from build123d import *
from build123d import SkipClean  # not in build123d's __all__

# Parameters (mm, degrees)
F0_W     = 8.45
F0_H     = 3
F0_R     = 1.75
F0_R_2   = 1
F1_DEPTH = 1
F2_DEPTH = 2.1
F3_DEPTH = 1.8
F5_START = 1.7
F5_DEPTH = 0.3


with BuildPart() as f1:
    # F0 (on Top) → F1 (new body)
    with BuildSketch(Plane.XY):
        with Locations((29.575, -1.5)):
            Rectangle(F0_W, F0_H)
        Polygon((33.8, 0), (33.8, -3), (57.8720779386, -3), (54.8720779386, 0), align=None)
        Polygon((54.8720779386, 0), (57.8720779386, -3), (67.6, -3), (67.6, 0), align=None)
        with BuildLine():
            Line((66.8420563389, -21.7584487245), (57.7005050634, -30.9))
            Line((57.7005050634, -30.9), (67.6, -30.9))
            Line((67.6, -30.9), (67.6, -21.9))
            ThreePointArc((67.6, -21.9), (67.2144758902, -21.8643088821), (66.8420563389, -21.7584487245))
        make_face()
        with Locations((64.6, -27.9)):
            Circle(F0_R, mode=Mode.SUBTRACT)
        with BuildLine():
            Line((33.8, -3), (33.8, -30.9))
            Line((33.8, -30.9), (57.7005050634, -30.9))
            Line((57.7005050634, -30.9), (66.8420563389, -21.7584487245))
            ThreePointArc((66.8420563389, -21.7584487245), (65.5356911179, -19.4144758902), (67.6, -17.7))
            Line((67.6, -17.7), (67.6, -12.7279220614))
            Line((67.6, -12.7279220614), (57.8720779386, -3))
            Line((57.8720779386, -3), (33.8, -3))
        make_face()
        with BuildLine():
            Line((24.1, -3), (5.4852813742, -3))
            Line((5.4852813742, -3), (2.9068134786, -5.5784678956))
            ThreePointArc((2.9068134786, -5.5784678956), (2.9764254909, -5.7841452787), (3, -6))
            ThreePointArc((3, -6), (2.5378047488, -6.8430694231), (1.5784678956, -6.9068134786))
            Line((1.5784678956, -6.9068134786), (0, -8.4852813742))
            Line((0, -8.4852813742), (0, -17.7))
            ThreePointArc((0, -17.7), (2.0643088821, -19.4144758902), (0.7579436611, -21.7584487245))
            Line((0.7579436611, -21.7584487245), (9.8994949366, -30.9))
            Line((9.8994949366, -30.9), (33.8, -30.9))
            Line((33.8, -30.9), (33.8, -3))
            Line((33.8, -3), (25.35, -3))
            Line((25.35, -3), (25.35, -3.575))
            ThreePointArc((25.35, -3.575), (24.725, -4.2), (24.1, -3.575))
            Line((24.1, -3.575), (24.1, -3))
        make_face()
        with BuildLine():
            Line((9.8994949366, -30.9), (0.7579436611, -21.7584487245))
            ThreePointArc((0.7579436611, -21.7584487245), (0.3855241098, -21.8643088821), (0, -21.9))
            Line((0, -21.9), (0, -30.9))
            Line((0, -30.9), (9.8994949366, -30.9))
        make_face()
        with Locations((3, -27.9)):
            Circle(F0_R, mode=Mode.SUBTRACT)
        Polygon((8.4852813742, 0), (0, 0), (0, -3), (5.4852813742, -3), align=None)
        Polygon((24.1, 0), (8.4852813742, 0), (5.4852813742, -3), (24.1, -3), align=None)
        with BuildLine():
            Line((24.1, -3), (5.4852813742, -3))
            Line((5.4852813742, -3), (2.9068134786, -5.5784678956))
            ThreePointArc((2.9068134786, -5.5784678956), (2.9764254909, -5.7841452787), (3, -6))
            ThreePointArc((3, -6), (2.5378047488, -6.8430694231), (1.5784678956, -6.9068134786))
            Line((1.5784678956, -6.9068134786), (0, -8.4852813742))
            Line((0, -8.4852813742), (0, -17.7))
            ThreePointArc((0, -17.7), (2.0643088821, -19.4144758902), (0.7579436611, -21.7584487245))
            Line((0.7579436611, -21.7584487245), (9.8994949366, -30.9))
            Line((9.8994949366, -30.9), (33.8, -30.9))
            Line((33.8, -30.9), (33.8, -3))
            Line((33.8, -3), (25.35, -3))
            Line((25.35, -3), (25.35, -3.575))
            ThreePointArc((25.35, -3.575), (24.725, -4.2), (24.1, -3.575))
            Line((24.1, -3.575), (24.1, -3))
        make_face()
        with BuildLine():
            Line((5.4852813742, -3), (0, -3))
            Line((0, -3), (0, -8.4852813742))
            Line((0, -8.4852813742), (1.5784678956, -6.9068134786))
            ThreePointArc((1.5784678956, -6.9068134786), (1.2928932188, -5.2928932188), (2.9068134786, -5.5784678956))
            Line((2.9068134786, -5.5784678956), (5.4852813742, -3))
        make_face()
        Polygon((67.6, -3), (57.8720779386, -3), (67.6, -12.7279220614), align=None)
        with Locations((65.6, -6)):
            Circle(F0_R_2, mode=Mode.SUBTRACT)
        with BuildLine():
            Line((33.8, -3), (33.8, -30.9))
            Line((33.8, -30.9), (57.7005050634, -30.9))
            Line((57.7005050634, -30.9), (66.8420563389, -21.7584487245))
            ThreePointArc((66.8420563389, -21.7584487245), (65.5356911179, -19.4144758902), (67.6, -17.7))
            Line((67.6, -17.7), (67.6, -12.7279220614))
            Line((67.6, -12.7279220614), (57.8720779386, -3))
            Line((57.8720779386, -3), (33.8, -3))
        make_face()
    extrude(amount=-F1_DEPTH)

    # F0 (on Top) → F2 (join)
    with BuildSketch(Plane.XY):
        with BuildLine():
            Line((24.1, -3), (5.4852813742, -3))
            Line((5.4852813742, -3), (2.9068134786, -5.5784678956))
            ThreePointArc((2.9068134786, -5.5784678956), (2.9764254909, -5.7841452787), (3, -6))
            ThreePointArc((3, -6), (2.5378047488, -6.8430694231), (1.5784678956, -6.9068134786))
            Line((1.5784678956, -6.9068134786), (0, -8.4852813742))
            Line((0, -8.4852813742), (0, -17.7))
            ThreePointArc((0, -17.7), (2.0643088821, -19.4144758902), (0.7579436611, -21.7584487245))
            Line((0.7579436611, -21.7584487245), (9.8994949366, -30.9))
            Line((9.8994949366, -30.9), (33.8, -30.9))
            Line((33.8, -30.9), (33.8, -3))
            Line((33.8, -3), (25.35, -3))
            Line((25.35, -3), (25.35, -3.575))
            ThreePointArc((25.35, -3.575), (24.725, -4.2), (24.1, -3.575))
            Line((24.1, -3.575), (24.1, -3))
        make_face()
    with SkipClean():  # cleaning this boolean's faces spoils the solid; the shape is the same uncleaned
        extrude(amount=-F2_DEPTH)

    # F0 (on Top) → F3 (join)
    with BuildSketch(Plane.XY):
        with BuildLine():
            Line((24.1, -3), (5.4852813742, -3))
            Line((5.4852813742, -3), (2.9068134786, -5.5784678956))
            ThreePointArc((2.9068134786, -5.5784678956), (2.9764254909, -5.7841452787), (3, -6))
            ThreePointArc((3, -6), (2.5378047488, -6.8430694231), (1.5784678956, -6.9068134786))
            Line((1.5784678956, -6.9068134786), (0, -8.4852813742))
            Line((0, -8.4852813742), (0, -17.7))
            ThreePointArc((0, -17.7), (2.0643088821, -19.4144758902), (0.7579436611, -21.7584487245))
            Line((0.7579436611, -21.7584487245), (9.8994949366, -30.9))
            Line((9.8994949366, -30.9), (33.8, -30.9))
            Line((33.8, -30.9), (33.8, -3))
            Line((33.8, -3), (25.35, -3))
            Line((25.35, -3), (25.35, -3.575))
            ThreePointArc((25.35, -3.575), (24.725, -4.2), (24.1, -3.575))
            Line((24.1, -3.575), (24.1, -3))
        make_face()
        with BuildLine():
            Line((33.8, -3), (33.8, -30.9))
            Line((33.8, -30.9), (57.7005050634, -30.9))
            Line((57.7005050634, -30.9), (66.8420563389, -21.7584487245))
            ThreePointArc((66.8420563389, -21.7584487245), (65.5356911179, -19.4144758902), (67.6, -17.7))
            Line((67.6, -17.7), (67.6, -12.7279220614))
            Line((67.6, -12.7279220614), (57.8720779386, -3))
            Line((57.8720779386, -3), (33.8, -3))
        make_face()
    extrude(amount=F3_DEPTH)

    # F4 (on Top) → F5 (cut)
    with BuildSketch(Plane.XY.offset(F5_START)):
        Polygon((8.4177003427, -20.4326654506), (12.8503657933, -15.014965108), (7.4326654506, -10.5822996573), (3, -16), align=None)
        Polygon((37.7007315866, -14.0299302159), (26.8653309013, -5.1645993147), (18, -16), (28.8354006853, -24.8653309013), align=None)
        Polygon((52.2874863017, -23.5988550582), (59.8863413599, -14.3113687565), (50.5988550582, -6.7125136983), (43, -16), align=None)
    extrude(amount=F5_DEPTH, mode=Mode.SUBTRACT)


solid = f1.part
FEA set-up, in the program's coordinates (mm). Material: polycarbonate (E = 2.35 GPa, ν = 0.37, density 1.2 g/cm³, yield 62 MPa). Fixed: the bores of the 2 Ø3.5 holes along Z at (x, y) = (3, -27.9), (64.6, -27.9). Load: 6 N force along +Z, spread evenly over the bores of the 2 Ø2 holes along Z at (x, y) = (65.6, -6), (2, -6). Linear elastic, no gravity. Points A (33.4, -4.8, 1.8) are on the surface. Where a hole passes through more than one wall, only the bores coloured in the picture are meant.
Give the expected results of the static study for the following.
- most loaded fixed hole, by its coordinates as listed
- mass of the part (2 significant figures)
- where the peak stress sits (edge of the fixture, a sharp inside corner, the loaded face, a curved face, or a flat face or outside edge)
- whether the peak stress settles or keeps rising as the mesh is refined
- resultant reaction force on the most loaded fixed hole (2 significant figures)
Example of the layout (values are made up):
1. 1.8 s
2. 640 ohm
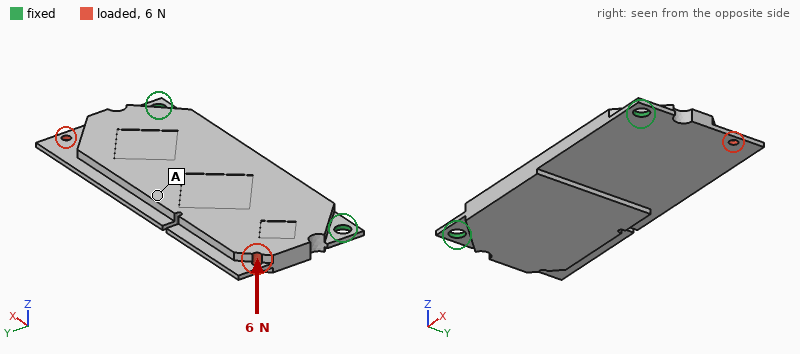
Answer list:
1. (3, -27.9)
2. 7.2 g
3. edge of the fixture
4. keeps rising
5. 5.8 N
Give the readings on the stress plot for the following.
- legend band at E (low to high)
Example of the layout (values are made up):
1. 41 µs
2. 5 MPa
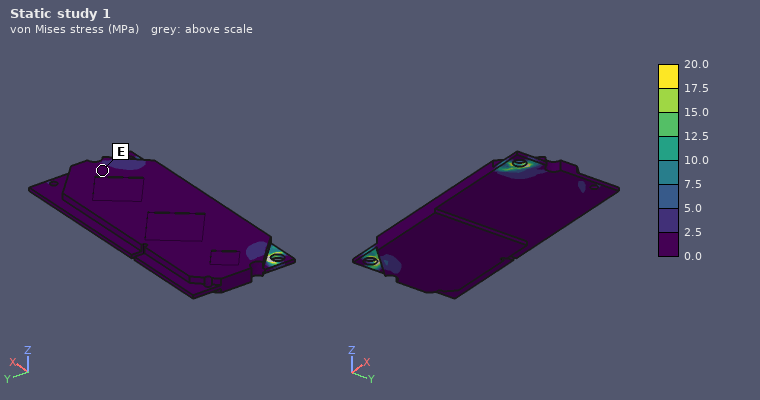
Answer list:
1. 0.0 to 2.5 MPa
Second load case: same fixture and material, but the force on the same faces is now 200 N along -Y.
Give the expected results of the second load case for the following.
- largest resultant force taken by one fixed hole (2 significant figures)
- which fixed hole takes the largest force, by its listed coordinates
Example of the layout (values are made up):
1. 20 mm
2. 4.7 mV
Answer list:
1. 140 N
2. (3, -27.9)
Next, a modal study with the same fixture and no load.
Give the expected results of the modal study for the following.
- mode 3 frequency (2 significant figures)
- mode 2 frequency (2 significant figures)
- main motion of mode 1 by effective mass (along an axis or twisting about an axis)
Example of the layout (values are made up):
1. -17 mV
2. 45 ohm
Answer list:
1. 1100 Hz
2. 890 Hz
3. along Z
